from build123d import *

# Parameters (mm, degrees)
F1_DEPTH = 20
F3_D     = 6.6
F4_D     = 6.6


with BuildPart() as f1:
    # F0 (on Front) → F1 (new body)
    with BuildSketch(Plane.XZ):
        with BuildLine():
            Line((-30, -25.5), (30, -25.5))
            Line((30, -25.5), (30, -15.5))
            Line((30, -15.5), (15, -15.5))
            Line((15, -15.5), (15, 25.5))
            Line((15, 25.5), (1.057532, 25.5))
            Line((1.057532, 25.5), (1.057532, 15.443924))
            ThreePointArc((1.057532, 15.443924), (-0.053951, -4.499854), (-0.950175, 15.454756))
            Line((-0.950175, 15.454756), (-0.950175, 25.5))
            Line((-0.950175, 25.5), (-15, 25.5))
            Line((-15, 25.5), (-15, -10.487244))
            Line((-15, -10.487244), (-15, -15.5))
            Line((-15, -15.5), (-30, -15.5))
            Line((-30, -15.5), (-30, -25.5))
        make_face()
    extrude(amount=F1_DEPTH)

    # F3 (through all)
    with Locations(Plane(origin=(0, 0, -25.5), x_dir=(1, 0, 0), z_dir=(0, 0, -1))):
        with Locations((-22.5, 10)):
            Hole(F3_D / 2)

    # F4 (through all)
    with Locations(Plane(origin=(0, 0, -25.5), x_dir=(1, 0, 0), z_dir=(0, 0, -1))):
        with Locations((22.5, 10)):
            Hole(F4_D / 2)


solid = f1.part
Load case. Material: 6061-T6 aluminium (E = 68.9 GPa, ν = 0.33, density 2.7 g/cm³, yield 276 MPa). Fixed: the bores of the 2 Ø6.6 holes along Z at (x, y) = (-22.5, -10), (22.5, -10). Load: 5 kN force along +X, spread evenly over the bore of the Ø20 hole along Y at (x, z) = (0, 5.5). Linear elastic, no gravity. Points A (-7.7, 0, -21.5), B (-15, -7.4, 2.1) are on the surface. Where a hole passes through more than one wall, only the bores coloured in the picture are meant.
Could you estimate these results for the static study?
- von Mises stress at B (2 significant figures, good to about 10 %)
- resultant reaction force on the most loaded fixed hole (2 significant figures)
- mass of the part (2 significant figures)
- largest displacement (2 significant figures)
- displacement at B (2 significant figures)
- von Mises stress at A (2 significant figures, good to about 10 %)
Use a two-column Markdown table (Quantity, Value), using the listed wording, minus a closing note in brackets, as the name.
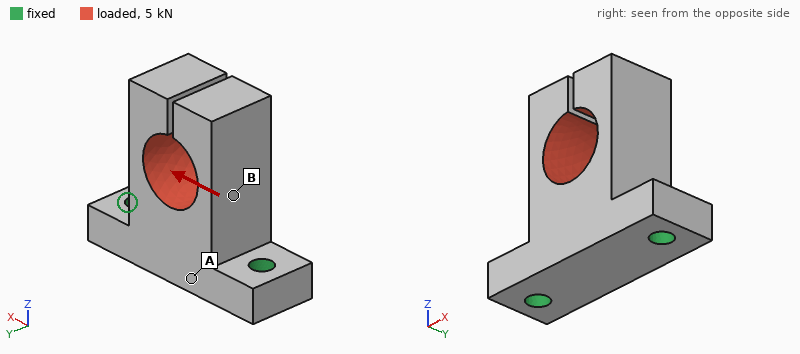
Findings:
| Quantity | Value |
|---|---|
| von Mises stress at B | 98 MPa |
| resultant reaction force on the most loaded fixed hole | 4.3 kN |
| mass of the part | 79 g |
| largest displacement | 0.24 mm |
| displacement at B | 0.050 mm |
| von Mises stress at A | 13 MPa |
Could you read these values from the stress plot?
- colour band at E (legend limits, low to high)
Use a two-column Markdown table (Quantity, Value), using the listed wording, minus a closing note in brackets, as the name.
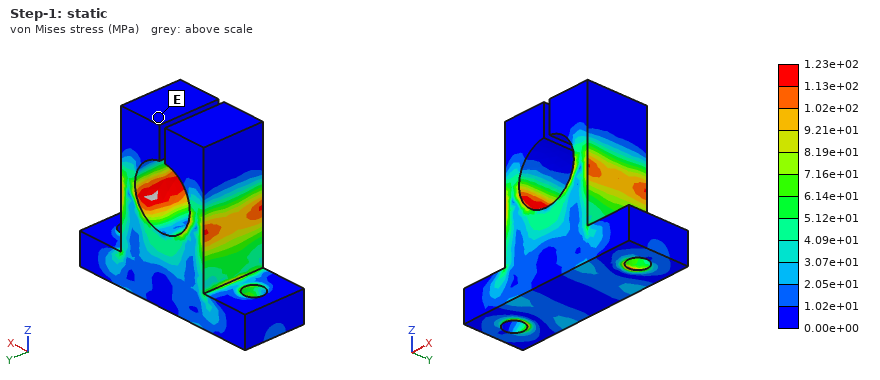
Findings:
| Quantity | Value |
|---|---|
| colour band at E | 0.00e+00 to 1.02e+01 MPa |
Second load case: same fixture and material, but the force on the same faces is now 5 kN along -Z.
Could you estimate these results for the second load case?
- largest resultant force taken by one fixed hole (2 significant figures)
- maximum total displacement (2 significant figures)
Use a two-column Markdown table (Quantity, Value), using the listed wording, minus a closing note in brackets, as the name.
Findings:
| Quantity | Value |
|---|---|
| largest resultant force taken by one fixed hole | 2.7 kN |
| maximum total displacement | 0.14 mm |
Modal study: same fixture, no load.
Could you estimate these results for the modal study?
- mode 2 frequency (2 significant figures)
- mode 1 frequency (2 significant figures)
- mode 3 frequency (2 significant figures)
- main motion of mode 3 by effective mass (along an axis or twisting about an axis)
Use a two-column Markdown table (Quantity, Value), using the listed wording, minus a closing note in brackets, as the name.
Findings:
| Quantity | Value |
|---|---|
| mode 2 frequency | 3300 Hz |
| mode 1 frequency | 3300 Hz |
| mode 3 frequency | 3500 Hz |
| main motion of mode 3 by effective mass | along Y |
